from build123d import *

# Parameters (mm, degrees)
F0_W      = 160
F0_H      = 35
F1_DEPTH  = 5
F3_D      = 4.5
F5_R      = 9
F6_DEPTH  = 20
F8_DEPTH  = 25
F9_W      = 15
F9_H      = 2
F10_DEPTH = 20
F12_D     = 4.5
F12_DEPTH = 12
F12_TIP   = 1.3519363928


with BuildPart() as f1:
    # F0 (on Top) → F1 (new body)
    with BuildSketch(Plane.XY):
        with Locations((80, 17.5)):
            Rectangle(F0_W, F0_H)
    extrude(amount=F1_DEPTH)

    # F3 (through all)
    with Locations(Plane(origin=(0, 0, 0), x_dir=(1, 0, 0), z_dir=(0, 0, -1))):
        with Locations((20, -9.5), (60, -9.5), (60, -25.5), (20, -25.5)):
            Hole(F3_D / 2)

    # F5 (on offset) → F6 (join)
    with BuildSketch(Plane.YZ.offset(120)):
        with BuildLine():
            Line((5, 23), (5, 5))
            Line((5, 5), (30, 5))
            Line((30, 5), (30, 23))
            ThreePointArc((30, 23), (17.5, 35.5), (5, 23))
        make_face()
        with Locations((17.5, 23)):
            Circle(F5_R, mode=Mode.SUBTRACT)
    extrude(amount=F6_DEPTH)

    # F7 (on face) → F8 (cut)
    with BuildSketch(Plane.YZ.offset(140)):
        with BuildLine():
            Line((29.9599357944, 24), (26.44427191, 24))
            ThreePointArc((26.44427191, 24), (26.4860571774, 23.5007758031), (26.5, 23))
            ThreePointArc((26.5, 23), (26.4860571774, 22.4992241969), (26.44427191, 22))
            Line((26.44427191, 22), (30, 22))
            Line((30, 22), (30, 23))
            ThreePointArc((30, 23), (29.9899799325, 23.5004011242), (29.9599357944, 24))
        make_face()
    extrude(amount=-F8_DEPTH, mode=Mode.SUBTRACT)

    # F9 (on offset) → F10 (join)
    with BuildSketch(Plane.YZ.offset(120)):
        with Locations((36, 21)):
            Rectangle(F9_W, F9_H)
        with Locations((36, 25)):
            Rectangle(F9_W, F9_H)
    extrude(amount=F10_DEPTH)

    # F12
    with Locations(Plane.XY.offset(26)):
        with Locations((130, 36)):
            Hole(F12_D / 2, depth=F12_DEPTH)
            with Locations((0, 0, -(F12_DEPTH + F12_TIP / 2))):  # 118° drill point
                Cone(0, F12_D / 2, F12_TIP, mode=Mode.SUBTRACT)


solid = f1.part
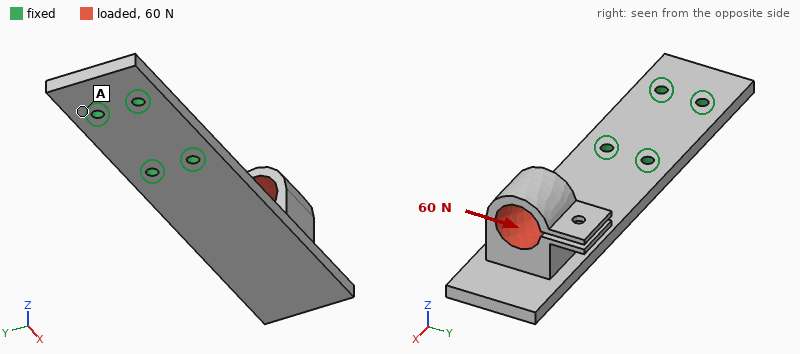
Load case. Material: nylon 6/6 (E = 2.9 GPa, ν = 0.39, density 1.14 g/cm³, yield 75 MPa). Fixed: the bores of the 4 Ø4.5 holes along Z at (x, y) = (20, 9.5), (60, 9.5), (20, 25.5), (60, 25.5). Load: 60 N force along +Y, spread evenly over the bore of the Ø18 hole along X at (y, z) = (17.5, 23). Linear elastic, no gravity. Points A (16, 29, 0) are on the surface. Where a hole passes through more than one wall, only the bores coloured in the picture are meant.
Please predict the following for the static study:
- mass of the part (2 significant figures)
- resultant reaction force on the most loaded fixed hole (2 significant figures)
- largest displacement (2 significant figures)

43 g
180 N
1.8 mm
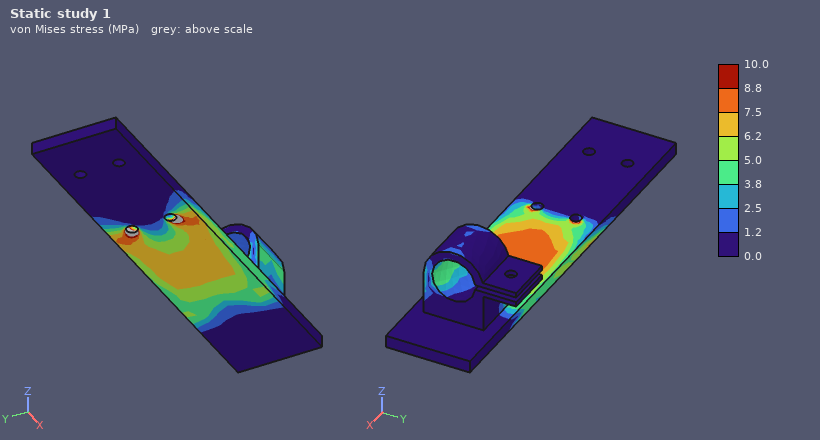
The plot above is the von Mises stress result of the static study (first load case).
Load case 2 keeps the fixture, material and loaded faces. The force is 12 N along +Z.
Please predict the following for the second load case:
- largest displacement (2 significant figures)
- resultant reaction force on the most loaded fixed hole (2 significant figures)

2.0 mm
7.1 N
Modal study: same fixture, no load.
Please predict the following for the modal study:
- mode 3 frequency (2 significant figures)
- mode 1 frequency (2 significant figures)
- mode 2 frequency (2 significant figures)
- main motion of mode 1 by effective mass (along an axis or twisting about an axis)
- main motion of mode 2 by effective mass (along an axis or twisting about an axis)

560 Hz
96 Hz
340 Hz
along Z
along Y
